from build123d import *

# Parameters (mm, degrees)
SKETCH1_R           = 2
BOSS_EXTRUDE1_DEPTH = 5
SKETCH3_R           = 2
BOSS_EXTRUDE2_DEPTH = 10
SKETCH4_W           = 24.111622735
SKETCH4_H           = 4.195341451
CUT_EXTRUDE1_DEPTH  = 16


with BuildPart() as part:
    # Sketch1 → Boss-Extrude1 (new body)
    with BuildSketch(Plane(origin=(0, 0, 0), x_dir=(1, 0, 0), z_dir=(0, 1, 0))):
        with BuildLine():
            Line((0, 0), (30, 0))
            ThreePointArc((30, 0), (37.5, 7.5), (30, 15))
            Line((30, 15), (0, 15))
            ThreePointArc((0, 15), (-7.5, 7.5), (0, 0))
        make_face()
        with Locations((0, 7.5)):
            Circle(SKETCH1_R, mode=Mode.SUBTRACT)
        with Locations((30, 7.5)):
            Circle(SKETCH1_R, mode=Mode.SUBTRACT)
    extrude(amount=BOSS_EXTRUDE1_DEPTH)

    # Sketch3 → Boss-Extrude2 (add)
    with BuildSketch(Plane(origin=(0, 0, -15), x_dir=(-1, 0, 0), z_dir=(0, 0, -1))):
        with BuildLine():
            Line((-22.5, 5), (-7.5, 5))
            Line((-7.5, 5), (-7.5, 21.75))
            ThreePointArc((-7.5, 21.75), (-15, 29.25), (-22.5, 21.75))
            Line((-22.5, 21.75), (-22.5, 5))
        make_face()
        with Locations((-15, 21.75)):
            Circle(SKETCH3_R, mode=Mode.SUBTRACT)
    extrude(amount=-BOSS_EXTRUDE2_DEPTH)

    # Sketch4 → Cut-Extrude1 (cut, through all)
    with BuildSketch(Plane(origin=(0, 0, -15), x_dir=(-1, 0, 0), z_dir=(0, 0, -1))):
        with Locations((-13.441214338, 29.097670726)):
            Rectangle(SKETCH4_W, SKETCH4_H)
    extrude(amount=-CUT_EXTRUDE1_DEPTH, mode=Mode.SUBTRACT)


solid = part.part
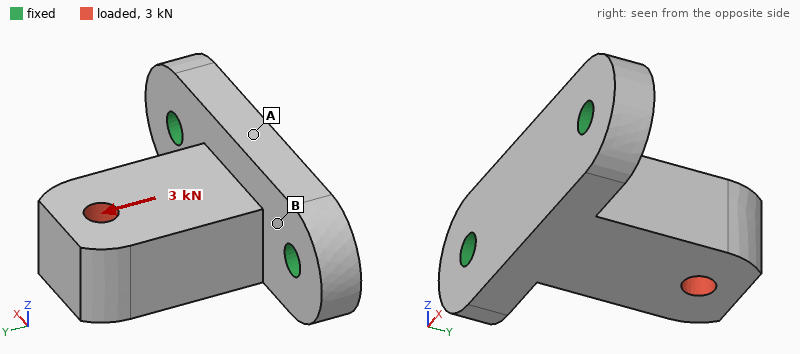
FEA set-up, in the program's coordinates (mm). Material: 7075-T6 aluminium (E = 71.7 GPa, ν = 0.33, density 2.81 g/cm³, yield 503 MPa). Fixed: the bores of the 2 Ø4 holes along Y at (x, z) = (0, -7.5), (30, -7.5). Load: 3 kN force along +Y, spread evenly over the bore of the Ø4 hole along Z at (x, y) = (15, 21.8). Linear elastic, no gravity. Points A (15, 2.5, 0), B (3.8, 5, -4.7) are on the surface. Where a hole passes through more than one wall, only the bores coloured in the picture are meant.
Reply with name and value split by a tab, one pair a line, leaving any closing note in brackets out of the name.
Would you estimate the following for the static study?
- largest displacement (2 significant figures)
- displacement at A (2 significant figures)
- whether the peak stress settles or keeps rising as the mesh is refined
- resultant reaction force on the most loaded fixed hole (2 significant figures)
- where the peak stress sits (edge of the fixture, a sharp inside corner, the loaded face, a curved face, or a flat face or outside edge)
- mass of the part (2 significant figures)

largest displacement	61 µm
displacement at A	9.5 µm
whether the peak stress settles or keeps rising as the mesh is refined	keeps rising
resultant reaction force on the most loaded fixed hole	1.6 kN
where the peak stress sits	edge of the fixture
mass of the part	17 g
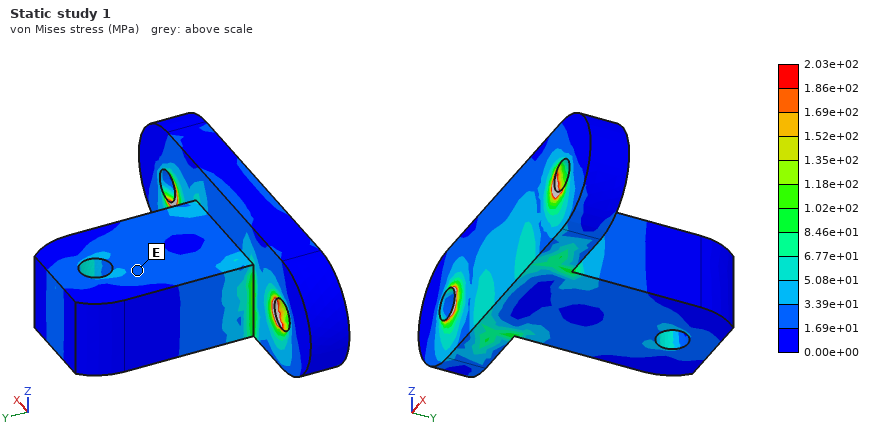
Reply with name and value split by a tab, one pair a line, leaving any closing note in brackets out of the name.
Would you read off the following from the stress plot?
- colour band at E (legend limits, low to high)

colour band at E	1.69e+01 to 3.39e+01 MPa
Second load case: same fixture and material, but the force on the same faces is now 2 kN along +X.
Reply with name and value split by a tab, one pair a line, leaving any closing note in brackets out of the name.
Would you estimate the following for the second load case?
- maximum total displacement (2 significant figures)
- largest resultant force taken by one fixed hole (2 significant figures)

maximum total displacement	89 µm
largest resultant force taken by one fixed hole	2.0 kN
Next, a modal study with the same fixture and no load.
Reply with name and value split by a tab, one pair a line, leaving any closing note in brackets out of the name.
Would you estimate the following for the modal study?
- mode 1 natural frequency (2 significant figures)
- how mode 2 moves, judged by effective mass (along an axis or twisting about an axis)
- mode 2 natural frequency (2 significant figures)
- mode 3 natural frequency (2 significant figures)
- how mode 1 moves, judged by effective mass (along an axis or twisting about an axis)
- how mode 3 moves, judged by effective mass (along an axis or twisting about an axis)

mode 1 natural frequency	5900 Hz
how mode 2 moves, judged by effective mass	along X
mode 2 natural frequency	12 kHz
mode 3 natural frequency	17 kHz
how mode 1 moves, judged by effective mass	along Z
how mode 3 moves, judged by effective mass	along Y
